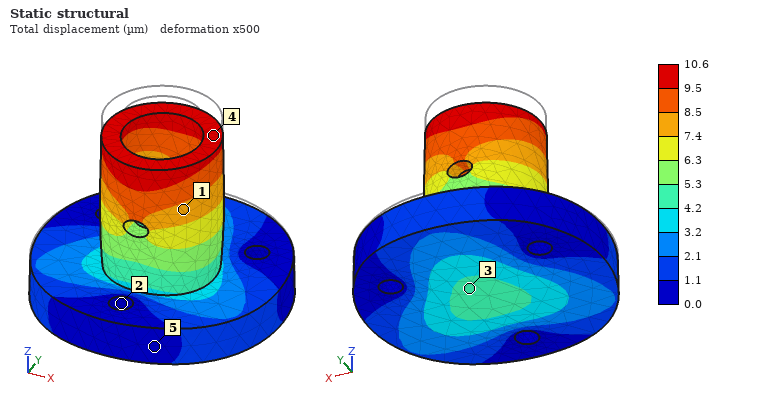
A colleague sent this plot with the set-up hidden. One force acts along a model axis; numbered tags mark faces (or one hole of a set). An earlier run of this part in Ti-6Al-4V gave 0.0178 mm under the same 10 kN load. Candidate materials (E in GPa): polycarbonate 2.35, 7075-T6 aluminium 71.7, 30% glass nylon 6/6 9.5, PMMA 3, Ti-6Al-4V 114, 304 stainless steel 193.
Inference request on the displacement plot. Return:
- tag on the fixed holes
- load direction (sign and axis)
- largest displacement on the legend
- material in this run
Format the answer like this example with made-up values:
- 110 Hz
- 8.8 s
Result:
- 2
- -Z
- 10.6 µm
- 304 stainless steel
